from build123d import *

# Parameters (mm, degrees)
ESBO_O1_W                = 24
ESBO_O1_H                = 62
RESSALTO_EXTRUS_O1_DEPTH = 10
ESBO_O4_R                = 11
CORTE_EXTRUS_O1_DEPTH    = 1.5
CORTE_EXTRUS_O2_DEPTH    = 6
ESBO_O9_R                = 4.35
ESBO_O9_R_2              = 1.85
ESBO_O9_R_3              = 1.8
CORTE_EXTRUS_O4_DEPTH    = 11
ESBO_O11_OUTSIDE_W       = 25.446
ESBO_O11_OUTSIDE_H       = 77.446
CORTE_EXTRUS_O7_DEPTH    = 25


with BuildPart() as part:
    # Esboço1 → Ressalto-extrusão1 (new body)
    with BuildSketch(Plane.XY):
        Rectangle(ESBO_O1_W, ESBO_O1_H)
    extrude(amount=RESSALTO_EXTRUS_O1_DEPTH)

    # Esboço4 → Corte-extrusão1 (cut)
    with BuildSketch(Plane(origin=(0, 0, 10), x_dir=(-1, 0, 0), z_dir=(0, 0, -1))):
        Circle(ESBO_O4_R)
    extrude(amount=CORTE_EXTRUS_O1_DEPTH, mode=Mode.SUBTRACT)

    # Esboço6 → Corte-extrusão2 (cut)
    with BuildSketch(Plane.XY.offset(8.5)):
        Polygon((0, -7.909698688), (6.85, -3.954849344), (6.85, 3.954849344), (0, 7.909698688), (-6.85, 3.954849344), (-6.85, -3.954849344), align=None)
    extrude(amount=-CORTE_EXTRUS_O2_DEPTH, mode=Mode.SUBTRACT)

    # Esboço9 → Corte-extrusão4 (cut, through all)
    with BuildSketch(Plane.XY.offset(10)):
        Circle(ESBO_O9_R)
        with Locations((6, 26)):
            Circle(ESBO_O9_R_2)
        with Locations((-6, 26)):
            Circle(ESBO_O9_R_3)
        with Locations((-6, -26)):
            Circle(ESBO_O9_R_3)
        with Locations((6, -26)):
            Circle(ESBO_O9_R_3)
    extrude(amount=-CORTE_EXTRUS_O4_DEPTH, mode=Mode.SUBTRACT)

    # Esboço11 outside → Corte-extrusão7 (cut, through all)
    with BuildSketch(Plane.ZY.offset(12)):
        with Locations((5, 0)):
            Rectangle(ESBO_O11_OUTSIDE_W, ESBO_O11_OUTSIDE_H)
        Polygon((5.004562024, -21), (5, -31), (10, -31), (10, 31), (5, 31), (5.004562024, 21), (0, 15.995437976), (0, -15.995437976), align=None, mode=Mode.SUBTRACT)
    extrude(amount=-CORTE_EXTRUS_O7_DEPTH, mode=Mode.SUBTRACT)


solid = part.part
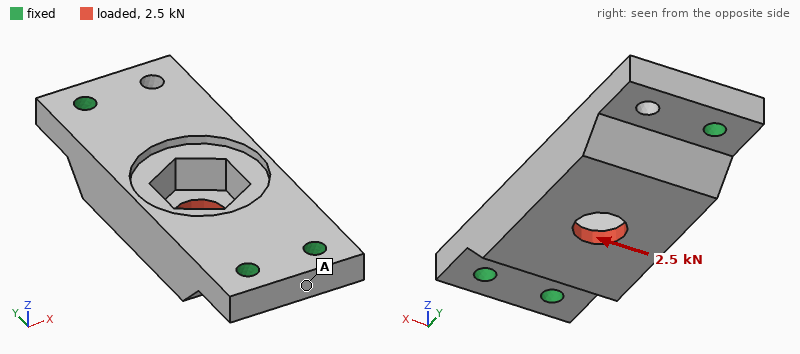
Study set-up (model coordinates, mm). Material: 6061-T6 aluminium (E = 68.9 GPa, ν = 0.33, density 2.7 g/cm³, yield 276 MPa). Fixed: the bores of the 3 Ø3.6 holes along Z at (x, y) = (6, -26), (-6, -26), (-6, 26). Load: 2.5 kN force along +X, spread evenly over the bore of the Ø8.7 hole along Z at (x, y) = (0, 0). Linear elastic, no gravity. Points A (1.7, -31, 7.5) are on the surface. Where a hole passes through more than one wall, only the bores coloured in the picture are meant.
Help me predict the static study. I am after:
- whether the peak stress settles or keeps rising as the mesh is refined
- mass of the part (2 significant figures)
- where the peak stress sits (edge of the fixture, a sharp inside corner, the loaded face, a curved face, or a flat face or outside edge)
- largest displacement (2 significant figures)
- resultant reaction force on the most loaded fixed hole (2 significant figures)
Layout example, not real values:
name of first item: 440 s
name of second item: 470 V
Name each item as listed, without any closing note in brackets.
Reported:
whether the peak stress settles or keeps rising as the mesh is refined: keeps rising
mass of the part: 27 g
where the peak stress sits: edge of the fixture
largest displacement: 45 µm
resultant reaction force on the most loaded fixed hole: 1.7 kN
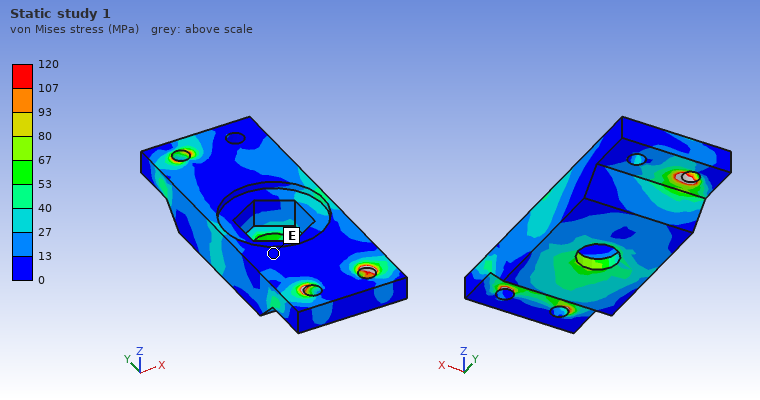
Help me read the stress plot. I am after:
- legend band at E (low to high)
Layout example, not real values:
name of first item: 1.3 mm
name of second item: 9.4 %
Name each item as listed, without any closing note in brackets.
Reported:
legend band at E: 0 to 13 MPa
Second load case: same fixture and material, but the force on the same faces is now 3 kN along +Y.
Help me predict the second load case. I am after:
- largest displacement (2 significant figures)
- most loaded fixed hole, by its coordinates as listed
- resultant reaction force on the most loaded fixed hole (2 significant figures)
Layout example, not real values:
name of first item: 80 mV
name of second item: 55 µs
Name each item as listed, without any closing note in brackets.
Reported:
largest displacement: 12 µm
most loaded fixed hole, by its coordinates as listed: (-6, 26)
resultant reaction force on the most loaded fixed hole: 1.3 kN
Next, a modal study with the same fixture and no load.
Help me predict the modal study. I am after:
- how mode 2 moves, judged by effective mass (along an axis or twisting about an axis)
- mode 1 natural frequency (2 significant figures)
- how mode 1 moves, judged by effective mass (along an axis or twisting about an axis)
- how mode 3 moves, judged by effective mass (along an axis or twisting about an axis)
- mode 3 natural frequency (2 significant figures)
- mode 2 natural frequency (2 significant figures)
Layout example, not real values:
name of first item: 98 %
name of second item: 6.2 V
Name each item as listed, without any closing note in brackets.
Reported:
how mode 2 moves, judged by effective mass: along Z
mode 1 natural frequency: 9000 Hz
how mode 1 moves, judged by effective mass: along Z
how mode 3 moves, judged by effective mass: along X
mode 3 natural frequency: 18 kHz
mode 2 natural frequency: 13 kHz
